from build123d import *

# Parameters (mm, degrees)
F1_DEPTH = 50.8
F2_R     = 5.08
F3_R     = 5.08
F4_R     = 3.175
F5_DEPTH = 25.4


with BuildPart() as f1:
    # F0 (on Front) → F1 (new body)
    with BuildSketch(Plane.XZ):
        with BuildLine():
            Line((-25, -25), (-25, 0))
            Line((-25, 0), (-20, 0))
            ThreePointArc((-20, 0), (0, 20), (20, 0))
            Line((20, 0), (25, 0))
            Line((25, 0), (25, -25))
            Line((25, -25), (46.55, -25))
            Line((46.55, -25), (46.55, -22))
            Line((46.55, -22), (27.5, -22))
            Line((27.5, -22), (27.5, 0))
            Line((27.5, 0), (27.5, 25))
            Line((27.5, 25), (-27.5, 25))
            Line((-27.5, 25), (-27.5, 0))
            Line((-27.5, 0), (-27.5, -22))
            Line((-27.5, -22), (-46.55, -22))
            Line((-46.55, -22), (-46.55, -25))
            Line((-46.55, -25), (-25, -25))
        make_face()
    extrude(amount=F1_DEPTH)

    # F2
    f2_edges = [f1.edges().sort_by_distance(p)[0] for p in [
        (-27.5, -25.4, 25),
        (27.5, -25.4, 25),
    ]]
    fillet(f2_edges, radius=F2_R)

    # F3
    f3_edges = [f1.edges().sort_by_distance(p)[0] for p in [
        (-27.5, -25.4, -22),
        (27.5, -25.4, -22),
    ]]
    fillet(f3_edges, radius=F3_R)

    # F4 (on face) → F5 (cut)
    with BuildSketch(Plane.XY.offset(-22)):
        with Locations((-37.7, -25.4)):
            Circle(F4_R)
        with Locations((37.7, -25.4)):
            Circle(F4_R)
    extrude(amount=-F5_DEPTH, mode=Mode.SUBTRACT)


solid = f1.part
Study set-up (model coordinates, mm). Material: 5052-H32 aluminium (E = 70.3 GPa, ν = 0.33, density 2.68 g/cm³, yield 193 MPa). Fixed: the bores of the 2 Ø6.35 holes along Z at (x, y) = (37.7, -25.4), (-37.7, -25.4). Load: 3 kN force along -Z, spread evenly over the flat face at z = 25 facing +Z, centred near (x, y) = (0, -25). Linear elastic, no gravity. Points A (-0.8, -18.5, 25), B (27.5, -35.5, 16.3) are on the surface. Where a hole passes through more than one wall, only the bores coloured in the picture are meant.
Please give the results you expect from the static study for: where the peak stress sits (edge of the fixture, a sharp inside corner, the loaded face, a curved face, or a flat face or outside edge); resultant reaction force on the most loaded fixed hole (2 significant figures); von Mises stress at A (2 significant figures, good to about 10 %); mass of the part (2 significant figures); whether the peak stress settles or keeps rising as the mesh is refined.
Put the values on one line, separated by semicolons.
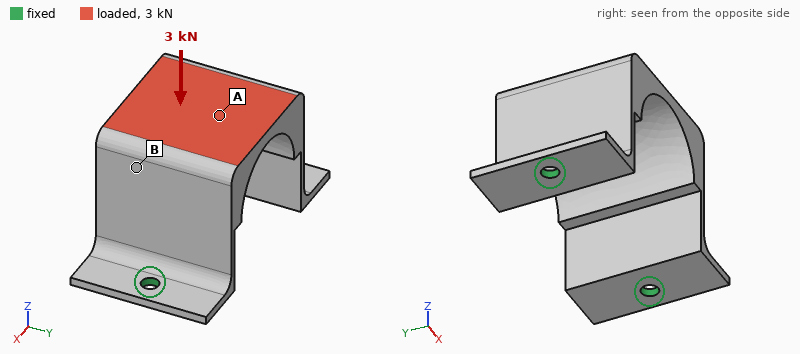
edge of the fixture; 1.6 kN; 28 MPa; 130 g; keeps rising
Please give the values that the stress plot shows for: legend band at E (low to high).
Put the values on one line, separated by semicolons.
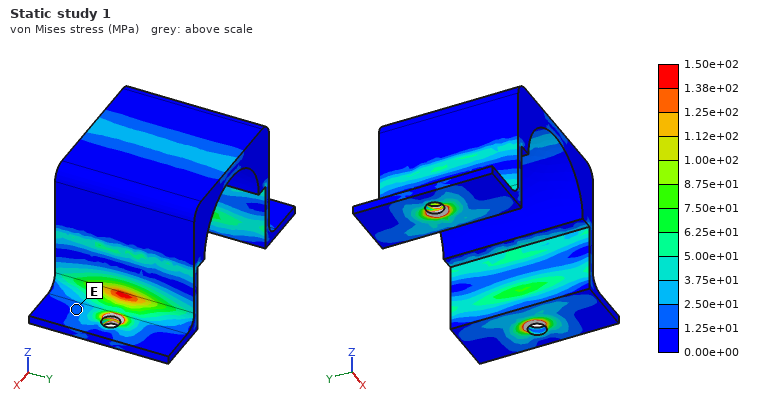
1.25e+01 to 2.50e+01 MPa
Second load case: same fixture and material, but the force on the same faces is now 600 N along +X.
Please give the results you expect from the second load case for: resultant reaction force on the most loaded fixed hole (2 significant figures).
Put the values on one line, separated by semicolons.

500 N
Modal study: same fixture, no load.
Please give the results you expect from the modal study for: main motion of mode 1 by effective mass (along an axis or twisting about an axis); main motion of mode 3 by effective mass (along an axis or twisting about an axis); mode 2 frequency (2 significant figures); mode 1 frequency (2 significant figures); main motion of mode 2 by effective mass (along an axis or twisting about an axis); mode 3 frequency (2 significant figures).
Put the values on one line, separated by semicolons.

along Y; twisting about Z; 1300 Hz; 600 Hz; along X; 2300 Hz
